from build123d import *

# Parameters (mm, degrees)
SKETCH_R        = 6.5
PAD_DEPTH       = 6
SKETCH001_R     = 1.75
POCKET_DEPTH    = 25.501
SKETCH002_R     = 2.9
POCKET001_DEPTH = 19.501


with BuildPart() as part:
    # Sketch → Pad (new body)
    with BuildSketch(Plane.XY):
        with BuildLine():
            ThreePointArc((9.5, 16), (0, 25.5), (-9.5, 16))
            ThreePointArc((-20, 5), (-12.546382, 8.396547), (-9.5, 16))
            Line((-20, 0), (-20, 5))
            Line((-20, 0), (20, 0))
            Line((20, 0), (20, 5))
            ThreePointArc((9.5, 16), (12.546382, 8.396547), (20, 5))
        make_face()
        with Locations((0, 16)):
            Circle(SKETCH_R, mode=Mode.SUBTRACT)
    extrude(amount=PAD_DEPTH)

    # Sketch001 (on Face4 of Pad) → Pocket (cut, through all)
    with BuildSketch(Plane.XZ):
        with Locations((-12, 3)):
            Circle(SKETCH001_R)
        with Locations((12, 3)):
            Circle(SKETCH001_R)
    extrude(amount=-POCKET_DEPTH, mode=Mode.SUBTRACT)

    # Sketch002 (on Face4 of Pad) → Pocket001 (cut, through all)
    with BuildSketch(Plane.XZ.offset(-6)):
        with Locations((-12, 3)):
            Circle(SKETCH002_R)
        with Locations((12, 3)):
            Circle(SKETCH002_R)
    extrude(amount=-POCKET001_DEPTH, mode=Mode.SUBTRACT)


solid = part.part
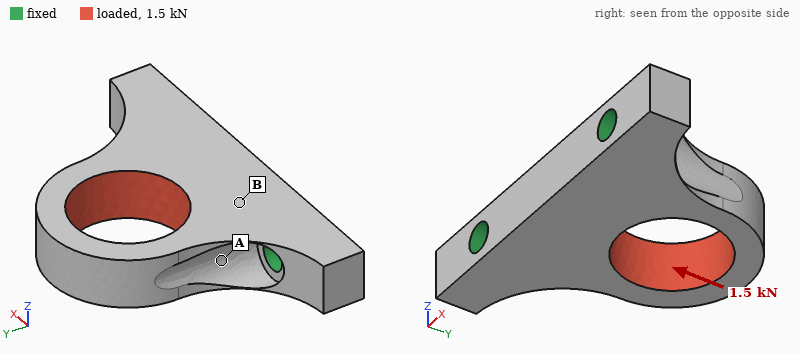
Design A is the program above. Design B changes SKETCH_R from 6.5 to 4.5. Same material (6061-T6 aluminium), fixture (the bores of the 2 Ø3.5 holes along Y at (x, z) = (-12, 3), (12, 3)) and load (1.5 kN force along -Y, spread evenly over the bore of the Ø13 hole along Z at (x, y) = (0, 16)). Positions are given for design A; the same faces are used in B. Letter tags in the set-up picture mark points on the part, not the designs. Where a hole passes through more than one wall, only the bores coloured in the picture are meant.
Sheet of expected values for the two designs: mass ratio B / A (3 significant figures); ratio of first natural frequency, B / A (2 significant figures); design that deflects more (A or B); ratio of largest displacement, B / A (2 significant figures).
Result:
1.16
0.91
A
0.57
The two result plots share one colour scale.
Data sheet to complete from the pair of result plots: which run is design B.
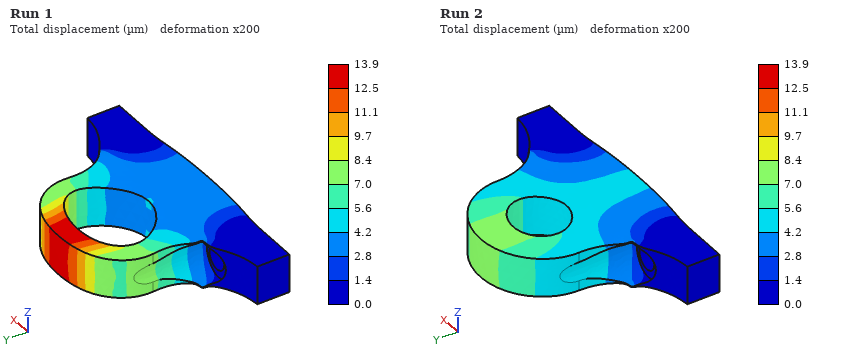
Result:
Run 2
